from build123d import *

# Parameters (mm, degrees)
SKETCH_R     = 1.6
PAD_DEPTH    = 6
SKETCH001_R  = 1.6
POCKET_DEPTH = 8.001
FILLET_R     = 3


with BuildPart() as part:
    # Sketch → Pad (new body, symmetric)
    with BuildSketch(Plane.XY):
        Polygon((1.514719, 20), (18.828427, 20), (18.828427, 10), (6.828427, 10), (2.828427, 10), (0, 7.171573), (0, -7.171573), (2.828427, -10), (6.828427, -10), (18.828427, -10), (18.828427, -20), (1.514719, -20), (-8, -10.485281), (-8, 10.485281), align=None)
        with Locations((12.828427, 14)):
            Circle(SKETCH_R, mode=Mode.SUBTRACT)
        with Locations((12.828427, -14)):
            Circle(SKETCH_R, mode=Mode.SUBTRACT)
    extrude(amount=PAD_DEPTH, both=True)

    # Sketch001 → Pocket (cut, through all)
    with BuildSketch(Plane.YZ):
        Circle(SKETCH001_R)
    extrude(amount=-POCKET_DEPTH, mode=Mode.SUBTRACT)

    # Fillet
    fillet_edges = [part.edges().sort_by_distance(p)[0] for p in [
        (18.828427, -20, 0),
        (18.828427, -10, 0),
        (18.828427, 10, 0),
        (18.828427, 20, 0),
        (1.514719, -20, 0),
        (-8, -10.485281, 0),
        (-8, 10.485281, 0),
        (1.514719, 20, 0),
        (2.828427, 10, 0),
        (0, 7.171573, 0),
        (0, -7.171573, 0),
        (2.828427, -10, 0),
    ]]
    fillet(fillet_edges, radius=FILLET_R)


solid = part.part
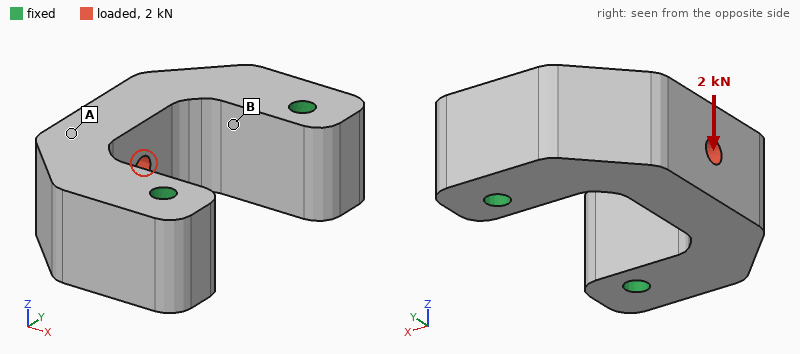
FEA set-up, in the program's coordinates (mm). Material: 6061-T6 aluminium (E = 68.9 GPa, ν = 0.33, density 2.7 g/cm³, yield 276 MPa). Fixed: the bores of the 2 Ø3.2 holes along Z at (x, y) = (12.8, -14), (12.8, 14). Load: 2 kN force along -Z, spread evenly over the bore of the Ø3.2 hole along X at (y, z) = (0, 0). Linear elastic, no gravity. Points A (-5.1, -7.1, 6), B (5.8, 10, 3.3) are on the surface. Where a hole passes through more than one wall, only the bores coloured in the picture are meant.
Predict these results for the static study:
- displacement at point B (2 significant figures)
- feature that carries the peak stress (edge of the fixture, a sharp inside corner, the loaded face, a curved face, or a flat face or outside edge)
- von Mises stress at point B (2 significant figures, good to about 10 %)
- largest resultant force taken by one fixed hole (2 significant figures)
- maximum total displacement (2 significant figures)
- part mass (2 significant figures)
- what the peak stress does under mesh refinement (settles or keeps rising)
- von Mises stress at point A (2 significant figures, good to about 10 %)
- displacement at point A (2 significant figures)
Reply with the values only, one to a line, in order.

8.9 µm
edge of the fixture
51 MPa
1.0 kN
44 µm
19 g
keeps rising
19 MPa
35 µm
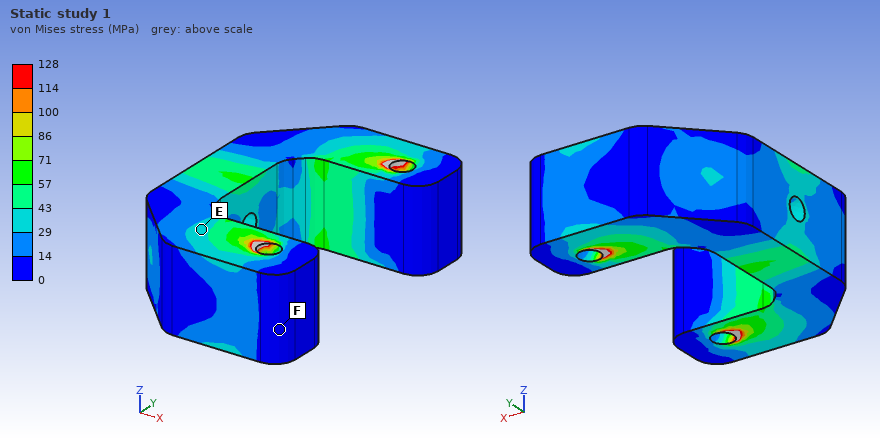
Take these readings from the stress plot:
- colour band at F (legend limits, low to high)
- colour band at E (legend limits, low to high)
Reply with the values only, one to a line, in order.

0 to 14 MPa
29 to 43 MPa
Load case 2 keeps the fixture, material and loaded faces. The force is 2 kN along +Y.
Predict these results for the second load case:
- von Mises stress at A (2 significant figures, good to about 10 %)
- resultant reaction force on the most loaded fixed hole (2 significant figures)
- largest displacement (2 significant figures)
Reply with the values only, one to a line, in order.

9.6 MPa
1.2 kN
21 µm
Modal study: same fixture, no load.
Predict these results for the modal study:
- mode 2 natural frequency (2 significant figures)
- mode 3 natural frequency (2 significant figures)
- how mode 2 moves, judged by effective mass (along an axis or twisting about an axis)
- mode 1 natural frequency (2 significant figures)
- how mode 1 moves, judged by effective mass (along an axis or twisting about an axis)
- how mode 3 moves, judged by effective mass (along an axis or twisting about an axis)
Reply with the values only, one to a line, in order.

17 kHz
27 kHz
along Y
15 kHz
along Z
twisting about X
